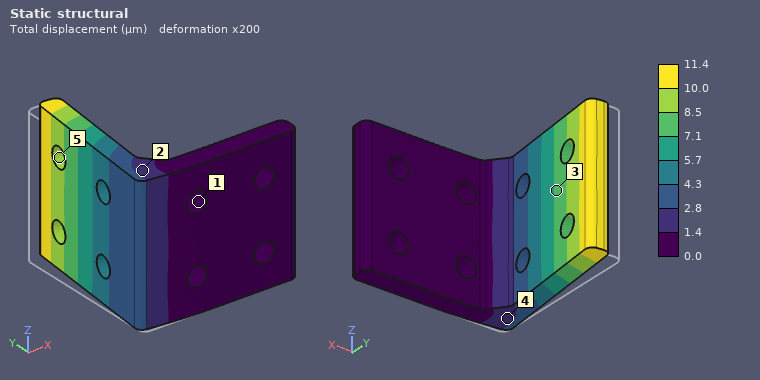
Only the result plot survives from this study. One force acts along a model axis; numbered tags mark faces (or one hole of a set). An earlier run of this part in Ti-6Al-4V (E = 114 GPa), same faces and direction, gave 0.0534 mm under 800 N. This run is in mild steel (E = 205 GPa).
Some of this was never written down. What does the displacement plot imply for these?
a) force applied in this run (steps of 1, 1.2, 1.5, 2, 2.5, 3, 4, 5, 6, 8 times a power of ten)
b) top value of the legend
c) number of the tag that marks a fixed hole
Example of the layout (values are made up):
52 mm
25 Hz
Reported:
300 N
11.4 µm
1
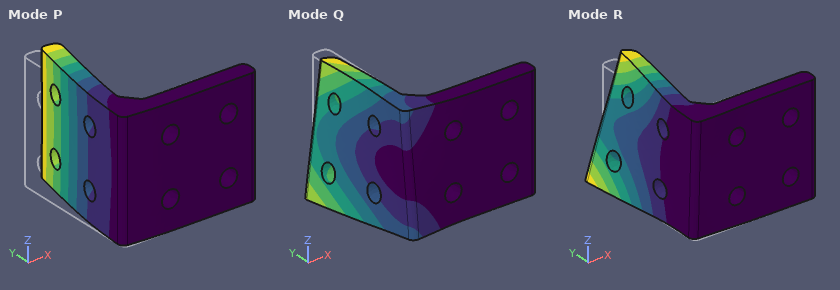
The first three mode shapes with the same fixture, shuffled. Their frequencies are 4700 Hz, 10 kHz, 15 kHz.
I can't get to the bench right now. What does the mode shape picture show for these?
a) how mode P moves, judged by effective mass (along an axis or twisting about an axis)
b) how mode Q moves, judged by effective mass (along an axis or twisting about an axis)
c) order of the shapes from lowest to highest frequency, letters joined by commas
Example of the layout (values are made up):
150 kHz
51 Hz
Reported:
along X
along Z
P, Q, R
